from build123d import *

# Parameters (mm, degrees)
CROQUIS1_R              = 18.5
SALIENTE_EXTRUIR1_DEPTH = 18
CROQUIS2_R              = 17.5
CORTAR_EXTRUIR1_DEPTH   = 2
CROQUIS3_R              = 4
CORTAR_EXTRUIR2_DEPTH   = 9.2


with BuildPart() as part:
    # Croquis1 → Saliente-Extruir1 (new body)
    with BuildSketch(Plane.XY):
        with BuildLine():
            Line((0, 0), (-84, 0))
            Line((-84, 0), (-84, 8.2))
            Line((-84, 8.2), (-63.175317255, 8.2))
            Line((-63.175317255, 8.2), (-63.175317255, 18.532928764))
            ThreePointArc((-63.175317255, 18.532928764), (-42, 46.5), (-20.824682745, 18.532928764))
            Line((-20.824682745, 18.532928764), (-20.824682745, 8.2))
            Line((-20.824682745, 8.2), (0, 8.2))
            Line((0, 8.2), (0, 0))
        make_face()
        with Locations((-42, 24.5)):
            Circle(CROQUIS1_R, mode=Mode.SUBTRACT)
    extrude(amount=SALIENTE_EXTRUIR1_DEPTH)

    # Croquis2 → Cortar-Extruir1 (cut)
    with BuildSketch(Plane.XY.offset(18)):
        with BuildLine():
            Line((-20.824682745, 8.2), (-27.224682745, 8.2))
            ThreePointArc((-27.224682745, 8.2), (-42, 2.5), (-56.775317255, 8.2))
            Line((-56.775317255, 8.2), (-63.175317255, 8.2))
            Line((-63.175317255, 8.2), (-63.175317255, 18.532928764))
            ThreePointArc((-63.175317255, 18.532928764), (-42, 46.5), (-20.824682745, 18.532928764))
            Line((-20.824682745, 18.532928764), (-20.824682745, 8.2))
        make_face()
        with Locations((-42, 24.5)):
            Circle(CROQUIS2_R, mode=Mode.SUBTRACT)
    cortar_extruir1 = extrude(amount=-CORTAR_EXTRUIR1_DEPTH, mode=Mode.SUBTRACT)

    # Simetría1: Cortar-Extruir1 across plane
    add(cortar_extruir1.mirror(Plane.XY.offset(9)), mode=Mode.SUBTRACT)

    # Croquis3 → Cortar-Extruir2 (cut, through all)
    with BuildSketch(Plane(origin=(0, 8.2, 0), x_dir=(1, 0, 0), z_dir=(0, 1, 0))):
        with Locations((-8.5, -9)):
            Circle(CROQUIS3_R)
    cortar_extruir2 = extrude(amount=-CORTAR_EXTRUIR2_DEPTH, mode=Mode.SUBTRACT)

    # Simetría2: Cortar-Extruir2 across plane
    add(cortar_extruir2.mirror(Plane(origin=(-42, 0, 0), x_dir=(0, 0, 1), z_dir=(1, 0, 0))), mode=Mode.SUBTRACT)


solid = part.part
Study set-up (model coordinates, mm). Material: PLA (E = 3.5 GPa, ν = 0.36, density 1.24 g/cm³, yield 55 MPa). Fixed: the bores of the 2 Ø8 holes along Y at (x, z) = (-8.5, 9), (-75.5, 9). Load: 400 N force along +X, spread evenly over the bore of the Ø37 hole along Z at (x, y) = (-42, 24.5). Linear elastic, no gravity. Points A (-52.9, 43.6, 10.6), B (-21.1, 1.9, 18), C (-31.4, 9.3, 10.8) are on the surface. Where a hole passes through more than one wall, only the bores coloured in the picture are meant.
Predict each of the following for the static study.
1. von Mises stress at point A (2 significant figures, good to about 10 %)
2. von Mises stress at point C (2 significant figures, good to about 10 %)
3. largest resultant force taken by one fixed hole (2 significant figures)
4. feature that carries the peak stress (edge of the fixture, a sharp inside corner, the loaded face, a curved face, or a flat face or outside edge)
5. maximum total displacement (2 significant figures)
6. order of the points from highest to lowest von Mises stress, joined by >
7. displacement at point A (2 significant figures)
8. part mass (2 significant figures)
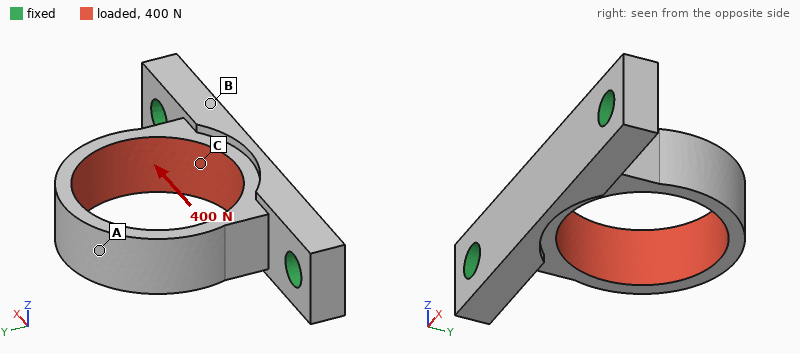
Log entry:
14 MPa
7.5 MPa
250 N
a curved face
0.91 mm
A > C > B
0.90 mm
20 g
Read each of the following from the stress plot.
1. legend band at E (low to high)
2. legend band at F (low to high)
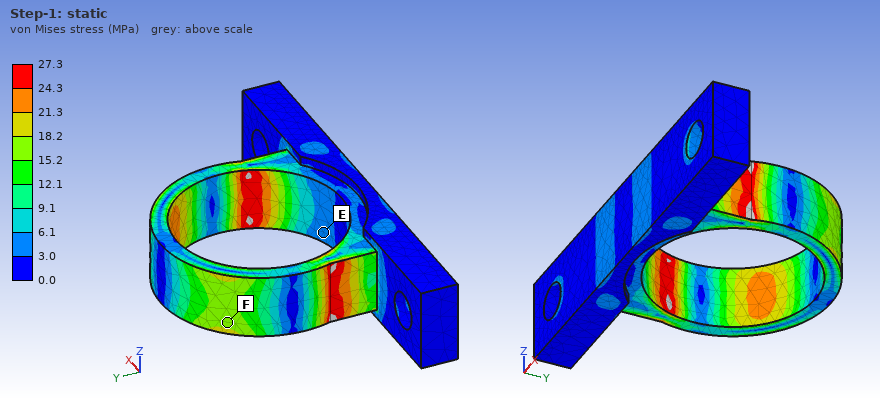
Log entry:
3.0 to 6.1 MPa
15.2 to 18.2 MPa
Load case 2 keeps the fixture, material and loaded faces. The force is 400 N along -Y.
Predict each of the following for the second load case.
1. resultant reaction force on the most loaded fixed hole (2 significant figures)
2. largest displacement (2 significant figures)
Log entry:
200 N
0.14 mm
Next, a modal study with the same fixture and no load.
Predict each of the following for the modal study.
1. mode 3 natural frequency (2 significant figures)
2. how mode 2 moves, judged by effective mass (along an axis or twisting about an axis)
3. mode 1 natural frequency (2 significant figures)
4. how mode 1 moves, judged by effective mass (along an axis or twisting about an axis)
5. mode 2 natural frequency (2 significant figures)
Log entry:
2700 Hz
along X
1200 Hz
along Z
1300 Hz
